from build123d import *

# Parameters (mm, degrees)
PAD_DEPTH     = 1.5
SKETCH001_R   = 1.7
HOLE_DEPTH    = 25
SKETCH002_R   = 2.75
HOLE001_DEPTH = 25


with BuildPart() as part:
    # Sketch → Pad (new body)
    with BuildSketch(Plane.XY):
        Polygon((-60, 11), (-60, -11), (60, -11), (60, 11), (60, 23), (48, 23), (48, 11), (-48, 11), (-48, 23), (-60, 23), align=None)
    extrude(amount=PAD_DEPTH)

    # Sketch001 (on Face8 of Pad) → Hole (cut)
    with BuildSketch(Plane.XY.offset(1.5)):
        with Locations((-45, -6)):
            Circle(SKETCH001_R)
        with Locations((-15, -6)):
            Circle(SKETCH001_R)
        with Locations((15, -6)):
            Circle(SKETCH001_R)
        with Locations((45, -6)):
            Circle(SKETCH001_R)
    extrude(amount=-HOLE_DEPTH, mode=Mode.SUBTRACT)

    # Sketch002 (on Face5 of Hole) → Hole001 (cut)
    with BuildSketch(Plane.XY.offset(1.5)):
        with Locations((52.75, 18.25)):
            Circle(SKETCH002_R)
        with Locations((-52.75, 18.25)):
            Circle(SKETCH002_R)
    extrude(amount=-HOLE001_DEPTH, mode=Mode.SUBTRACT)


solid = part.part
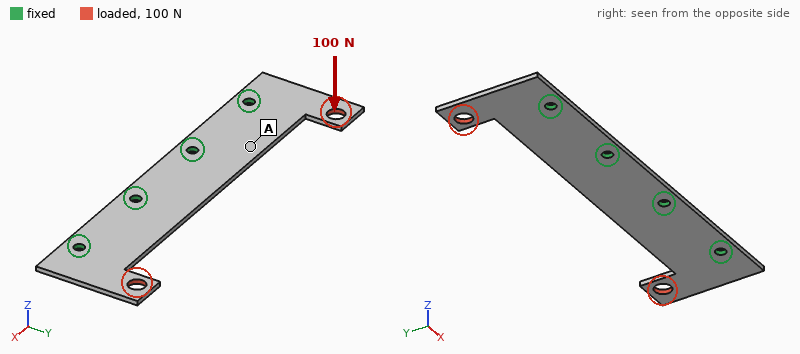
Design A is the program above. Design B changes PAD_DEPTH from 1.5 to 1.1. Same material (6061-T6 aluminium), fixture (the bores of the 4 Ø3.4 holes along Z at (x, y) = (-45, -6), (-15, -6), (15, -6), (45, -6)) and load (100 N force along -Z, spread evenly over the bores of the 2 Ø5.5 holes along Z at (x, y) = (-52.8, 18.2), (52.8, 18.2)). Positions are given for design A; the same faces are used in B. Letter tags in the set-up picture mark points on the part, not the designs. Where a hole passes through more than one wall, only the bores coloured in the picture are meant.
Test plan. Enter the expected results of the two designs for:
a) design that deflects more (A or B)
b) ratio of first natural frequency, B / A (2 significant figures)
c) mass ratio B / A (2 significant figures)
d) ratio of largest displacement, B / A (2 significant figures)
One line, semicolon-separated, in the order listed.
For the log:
B; 0.74; 0.73; 2.5
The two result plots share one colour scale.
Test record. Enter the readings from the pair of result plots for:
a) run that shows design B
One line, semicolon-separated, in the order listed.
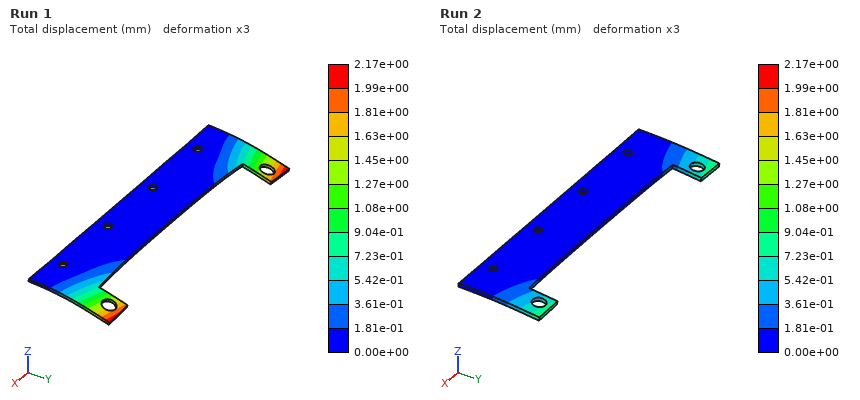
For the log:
Run 1
